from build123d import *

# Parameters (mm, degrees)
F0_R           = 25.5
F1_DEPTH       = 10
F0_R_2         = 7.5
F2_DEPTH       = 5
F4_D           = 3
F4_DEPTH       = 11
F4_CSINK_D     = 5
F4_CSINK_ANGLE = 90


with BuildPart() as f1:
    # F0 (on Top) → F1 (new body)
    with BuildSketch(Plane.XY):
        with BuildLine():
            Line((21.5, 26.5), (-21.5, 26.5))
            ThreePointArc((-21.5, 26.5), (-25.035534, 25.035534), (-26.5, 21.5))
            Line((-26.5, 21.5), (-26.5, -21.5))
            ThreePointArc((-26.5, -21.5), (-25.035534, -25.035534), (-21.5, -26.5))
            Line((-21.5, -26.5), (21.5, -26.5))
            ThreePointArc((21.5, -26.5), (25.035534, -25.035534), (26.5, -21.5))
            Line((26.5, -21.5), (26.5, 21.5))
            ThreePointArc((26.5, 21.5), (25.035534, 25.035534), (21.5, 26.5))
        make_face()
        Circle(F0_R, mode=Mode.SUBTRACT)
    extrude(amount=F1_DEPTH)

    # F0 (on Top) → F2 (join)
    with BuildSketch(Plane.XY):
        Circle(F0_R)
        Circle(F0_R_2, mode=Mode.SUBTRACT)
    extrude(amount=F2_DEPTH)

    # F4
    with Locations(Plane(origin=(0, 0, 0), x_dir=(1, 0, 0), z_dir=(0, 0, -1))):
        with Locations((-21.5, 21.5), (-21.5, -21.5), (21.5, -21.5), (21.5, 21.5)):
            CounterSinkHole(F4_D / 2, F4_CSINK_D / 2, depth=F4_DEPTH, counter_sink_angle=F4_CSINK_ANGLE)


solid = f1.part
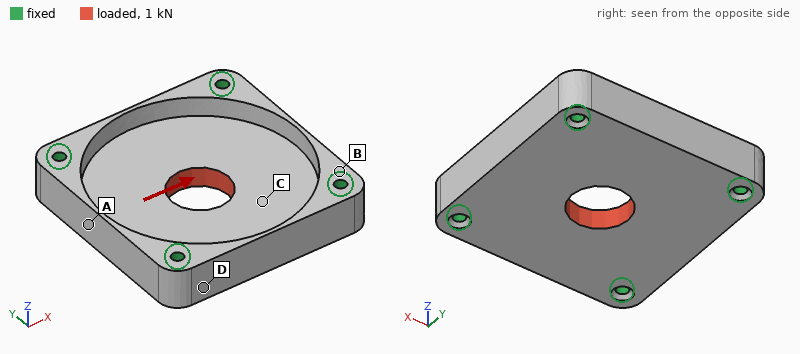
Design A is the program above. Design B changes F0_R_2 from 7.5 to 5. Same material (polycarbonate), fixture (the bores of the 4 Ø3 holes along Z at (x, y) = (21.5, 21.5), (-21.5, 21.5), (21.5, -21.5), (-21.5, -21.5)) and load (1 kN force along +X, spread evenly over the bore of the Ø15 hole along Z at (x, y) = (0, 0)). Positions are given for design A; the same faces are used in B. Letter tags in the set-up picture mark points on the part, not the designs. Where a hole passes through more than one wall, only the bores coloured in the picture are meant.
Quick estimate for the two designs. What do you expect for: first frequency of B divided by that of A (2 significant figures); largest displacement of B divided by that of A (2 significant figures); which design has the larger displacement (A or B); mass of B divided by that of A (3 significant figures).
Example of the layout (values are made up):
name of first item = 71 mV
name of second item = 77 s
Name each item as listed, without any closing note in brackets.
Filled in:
first frequency of B divided by that of A = 0.97
largest displacement of B divided by that of A = 1.1
which design has the larger displacement = B
mass of B divided by that of A = 1.03
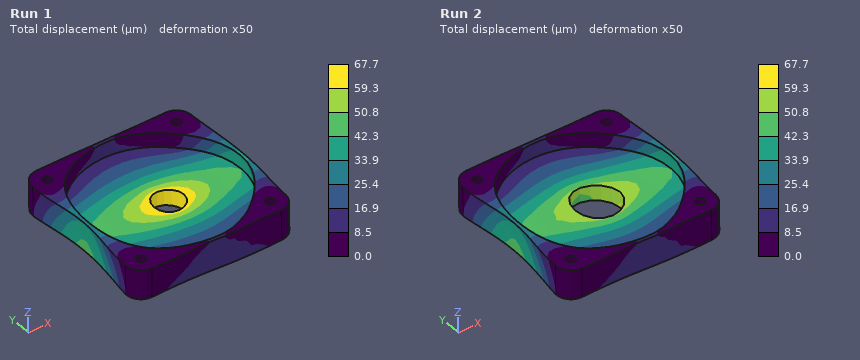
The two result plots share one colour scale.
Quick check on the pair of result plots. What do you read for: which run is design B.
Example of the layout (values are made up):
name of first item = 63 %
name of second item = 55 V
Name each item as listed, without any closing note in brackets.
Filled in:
which run is design B = Run 1
